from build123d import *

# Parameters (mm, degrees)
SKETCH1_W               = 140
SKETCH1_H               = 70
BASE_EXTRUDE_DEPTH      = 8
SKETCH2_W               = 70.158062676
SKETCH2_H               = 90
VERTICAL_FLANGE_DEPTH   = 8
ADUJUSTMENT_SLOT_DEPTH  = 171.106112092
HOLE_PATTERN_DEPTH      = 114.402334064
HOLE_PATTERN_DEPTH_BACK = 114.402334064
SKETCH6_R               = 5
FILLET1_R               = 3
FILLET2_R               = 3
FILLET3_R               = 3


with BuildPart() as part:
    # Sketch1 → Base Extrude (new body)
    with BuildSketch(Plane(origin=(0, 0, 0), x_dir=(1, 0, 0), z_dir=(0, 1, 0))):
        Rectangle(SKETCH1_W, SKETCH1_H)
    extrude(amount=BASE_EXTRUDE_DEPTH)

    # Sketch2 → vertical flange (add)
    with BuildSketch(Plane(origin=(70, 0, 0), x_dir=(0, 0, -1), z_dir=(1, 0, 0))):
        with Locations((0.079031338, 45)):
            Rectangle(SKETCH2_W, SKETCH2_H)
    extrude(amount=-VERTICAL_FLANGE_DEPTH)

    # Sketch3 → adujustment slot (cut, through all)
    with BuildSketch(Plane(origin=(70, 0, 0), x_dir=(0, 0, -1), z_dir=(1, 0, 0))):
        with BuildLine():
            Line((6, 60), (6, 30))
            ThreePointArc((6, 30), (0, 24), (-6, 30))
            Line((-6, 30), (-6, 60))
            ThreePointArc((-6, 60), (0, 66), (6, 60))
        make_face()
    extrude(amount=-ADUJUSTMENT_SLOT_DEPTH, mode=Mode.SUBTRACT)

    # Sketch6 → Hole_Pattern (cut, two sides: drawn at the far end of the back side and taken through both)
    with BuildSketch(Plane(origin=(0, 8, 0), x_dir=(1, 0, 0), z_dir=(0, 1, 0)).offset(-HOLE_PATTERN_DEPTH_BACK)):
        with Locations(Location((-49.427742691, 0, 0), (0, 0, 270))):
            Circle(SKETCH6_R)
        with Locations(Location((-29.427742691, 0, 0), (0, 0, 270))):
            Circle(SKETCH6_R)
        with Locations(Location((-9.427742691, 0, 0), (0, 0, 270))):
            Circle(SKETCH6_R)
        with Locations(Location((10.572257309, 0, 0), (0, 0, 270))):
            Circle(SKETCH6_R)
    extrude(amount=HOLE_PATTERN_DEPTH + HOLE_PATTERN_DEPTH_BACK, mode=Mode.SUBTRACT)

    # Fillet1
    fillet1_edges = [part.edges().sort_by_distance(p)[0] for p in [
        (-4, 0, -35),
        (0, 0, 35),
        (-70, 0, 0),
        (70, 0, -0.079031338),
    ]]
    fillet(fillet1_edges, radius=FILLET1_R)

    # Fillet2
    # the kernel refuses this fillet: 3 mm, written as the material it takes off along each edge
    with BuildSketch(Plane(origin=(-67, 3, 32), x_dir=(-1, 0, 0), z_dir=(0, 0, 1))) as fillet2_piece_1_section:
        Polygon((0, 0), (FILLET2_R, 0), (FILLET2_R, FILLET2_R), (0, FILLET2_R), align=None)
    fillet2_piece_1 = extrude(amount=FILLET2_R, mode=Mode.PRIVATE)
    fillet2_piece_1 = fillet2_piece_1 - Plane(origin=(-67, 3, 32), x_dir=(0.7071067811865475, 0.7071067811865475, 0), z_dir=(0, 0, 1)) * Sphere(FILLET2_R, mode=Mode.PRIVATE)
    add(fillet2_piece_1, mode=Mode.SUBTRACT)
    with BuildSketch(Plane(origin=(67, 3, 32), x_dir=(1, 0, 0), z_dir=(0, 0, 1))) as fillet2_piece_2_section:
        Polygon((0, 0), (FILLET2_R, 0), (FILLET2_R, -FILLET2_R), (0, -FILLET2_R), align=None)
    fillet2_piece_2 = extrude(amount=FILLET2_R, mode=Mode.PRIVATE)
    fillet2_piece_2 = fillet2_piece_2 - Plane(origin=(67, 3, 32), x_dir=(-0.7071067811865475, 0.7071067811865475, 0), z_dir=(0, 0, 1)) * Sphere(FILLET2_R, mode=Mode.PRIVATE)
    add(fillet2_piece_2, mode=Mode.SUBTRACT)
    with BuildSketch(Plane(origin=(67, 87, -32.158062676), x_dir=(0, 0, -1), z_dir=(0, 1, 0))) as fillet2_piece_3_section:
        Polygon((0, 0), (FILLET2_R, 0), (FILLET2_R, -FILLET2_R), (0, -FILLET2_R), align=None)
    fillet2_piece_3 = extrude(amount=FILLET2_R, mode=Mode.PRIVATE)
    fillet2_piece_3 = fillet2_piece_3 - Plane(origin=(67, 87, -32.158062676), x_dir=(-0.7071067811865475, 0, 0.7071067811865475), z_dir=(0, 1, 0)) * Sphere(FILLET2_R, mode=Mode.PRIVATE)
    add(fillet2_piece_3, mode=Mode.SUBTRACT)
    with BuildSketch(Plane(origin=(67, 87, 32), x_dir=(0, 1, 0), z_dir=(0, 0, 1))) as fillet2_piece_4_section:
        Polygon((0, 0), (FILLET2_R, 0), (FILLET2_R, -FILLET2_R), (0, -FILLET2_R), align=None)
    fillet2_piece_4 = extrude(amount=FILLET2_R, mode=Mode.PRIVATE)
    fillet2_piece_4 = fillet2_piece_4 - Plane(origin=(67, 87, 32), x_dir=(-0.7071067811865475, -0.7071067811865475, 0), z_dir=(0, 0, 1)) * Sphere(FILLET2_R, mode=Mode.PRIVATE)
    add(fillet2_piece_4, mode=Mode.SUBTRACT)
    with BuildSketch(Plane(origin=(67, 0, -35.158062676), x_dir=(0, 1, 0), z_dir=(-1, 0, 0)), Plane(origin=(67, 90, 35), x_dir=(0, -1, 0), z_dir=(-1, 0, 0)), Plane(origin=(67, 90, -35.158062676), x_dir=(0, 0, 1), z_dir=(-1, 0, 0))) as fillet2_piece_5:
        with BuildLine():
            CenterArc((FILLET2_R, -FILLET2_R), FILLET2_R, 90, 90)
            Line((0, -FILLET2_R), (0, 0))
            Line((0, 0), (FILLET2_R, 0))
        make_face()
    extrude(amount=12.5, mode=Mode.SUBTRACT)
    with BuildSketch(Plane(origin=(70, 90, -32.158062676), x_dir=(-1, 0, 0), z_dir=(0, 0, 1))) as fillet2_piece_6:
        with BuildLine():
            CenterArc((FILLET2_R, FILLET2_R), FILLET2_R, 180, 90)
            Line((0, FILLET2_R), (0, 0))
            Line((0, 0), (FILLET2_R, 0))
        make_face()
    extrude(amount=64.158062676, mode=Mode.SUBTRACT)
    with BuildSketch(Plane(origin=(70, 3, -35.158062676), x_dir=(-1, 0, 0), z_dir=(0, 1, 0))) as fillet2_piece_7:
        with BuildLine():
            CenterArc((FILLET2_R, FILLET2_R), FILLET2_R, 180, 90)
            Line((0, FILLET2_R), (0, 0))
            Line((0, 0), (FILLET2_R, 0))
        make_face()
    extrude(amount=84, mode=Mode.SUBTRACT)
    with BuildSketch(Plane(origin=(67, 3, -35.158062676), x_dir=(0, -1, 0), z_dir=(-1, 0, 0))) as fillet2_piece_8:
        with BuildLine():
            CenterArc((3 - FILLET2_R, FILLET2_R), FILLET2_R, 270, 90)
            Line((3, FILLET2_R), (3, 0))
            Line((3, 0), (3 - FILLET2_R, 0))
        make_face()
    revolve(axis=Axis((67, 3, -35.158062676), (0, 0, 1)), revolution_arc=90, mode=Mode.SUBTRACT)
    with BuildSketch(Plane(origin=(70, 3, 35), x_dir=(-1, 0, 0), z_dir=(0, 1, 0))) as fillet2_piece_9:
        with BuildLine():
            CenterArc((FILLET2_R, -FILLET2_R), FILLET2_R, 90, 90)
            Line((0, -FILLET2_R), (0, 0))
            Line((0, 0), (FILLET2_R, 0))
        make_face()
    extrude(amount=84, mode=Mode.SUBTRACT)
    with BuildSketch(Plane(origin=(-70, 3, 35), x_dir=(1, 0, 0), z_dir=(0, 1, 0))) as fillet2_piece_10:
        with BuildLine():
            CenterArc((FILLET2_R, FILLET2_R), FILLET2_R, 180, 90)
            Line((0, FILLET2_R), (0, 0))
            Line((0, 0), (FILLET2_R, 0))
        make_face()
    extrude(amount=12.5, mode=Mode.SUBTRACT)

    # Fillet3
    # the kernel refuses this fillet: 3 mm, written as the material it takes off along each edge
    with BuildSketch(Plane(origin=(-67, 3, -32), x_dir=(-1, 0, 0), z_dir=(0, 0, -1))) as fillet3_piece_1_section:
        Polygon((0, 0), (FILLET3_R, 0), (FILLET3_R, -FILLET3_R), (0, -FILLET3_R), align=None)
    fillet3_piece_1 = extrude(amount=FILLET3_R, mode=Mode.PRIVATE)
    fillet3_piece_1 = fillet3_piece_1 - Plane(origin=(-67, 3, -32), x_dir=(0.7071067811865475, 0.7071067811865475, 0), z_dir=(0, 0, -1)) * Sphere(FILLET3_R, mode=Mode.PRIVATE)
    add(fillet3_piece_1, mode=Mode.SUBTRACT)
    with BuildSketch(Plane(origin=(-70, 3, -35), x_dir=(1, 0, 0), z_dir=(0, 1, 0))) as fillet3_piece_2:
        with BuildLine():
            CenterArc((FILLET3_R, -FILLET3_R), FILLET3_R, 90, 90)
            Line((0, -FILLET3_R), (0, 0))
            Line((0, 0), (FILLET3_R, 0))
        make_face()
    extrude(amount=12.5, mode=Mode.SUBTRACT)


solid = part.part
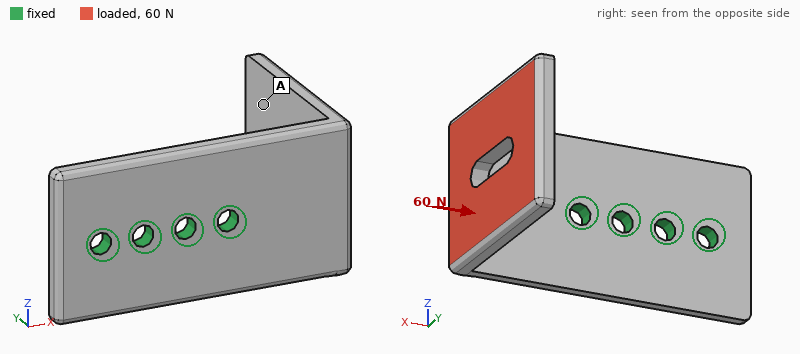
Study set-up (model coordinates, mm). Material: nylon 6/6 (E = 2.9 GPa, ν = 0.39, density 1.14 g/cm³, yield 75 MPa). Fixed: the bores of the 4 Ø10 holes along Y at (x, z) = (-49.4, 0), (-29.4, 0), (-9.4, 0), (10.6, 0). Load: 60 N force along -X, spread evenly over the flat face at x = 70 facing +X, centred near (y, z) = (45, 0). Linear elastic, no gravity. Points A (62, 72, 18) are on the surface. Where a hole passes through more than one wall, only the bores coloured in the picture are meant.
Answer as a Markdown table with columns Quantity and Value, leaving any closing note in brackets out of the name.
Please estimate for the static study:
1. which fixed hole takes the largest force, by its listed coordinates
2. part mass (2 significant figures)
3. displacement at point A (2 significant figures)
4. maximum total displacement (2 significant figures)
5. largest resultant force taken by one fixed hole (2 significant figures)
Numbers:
| Quantity | Value |
|---|---|
| which fixed hole takes the largest force, by its listed coordinates | (10.6, 0) |
| part mass | 130 g |
| displacement at point A | 1.4 mm |
| maximum total displacement | 1.8 mm |
| largest resultant force taken by one fixed hole | 60 N |
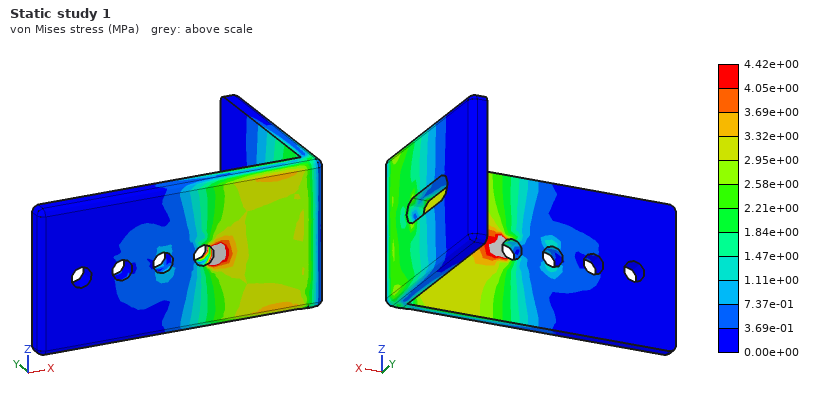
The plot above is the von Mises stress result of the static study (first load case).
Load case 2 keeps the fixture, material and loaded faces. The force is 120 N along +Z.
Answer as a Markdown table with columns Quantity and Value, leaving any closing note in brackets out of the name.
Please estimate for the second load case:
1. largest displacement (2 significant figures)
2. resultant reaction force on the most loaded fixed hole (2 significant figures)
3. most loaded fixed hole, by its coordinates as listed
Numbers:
| Quantity | Value |
|---|---|
| largest displacement | 1.8 mm |
| resultant reaction force on the most loaded fixed hole | 230 N |
| most loaded fixed hole, by its coordinates as listed | (10.6, 0) |
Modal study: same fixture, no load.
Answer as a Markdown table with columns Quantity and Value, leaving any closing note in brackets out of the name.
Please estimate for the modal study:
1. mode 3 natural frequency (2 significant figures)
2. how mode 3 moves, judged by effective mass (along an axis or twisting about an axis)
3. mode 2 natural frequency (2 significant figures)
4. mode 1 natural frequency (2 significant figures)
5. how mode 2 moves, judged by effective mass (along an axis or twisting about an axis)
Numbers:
| Quantity | Value |
|---|---|
| mode 3 natural frequency | 410 Hz |
| how mode 3 moves, judged by effective mass | along Y |
| mode 2 natural frequency | 200 Hz |
| mode 1 natural frequency | 140 Hz |
| how mode 2 moves, judged by effective mass | along Z |
